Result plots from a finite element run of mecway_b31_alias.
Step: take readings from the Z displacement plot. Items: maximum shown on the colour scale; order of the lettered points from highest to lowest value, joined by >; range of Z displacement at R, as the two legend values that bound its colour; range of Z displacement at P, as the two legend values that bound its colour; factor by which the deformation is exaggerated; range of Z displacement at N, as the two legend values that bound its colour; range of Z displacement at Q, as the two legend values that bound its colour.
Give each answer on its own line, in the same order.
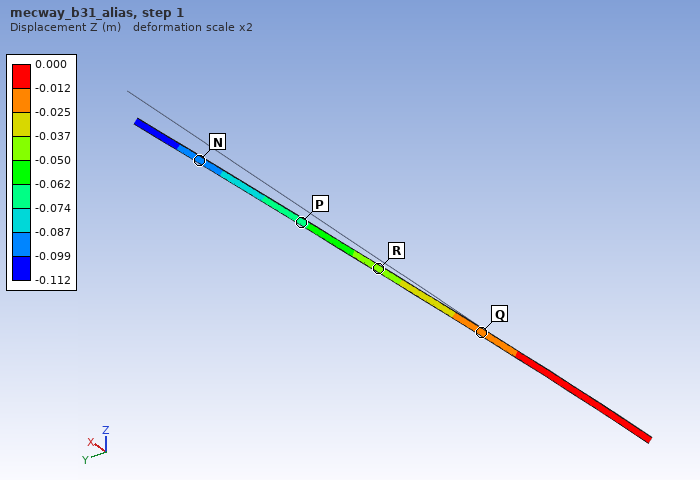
0.000 m
Q > R > P > N
-0.050 to -0.037 m
-0.074 to -0.062 m
2
-0.099 to -0.087 m
-0.025 to -0.012 m
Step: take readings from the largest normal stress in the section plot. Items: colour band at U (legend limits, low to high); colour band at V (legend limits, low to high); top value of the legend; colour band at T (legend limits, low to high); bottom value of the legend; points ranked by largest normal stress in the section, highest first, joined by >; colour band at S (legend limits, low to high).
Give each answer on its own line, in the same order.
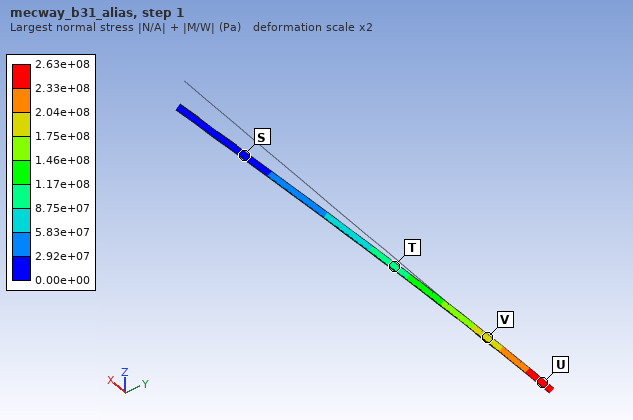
2.33e+08 to 2.63e+08 Pa
1.75e+08 to 2.04e+08 Pa
2.63e+08 Pa
8.75e+07 to 1.17e+08 Pa
0.00e+00 Pa
U > V > T > S
0.00e+00 to 2.92e+07 Pa
